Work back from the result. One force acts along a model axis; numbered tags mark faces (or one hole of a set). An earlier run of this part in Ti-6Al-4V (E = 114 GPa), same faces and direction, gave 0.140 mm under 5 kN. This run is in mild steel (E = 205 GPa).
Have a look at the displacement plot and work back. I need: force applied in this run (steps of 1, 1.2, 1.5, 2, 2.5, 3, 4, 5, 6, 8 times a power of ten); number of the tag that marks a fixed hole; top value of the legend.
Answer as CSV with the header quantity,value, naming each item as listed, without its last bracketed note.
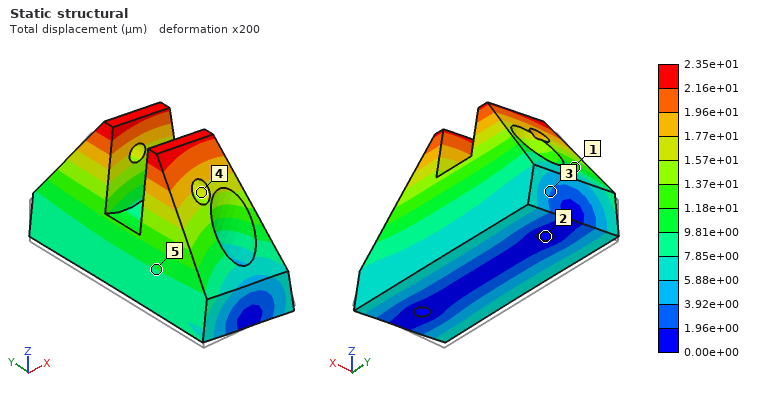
quantity,value
force applied in this run,1.5 kN
number of the tag that marks a fixed hole,2
top value of the legend,2.35e+01 µm
